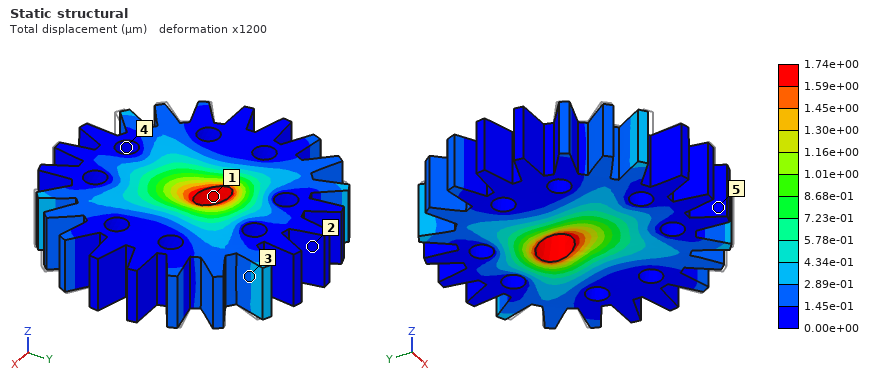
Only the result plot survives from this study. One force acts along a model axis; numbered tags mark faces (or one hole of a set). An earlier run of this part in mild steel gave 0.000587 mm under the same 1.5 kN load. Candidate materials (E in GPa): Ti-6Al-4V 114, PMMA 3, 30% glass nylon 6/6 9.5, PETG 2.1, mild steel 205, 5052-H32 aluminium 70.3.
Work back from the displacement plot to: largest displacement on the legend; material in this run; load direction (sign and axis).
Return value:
1.74e+00 µm
5052-H32 aluminium
+Y
